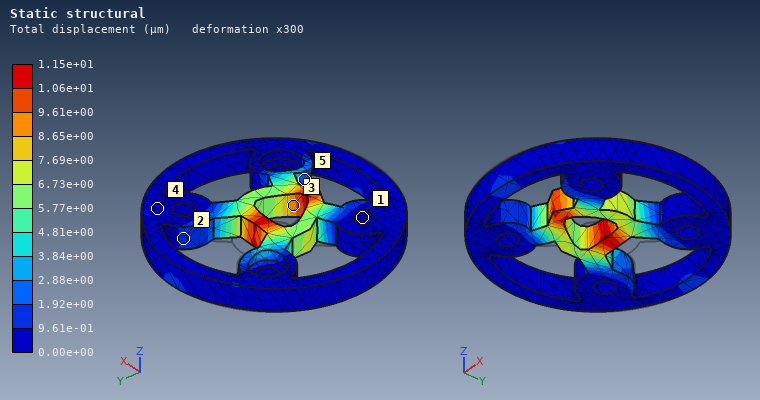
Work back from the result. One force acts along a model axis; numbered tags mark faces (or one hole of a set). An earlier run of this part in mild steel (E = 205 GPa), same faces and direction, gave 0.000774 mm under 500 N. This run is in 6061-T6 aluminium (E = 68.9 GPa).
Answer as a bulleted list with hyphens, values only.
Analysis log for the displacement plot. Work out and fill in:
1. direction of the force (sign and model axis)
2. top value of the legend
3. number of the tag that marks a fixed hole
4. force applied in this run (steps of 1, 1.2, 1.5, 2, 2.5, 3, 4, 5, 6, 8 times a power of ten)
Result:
- -Y
- 1.15e+01 µm
- 1
- 2.5 kN
